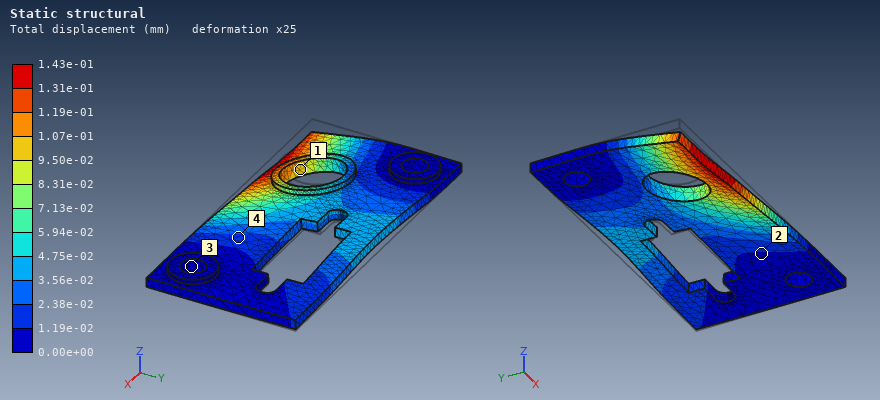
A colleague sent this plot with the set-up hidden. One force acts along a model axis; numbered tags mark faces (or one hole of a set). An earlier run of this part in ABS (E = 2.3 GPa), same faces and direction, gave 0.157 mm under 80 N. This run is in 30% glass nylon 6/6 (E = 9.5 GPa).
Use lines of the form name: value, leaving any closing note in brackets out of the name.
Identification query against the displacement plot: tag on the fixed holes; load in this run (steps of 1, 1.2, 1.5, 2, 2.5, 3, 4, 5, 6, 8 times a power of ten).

tag on the fixed holes: 3
load in this run: 300 N
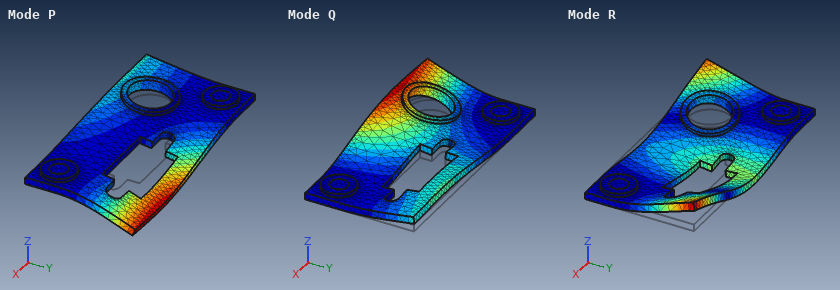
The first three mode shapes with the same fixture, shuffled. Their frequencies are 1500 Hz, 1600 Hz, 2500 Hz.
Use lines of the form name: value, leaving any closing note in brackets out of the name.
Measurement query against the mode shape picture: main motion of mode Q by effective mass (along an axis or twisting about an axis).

main motion of mode Q by effective mass: along Z
